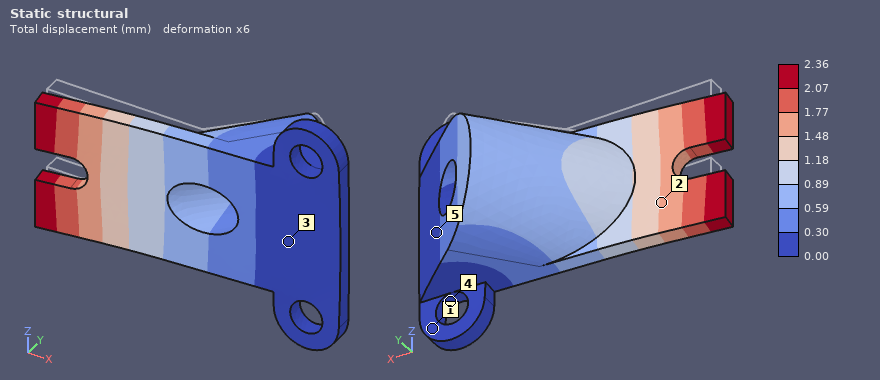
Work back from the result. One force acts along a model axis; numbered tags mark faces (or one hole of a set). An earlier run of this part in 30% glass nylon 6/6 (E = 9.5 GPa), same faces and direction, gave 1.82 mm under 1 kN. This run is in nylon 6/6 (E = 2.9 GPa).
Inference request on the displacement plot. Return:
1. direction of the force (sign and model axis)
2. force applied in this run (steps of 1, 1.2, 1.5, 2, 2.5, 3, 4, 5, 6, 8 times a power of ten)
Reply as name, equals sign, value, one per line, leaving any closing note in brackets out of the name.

direction of the force = -Y
force applied in this run = 400 N
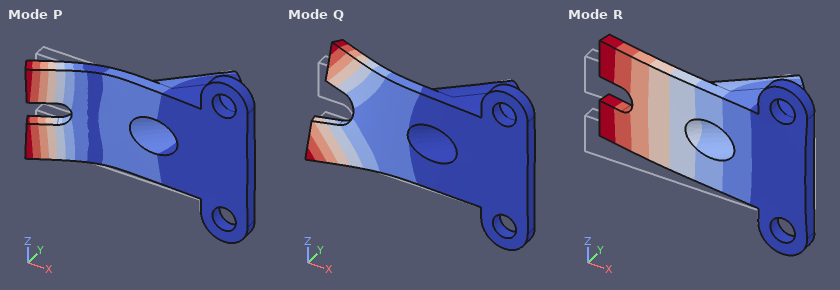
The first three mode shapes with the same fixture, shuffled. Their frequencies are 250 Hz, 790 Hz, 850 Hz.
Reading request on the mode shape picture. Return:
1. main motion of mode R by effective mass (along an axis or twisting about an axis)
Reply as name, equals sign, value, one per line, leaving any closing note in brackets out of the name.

main motion of mode R by effective mass = along Y
